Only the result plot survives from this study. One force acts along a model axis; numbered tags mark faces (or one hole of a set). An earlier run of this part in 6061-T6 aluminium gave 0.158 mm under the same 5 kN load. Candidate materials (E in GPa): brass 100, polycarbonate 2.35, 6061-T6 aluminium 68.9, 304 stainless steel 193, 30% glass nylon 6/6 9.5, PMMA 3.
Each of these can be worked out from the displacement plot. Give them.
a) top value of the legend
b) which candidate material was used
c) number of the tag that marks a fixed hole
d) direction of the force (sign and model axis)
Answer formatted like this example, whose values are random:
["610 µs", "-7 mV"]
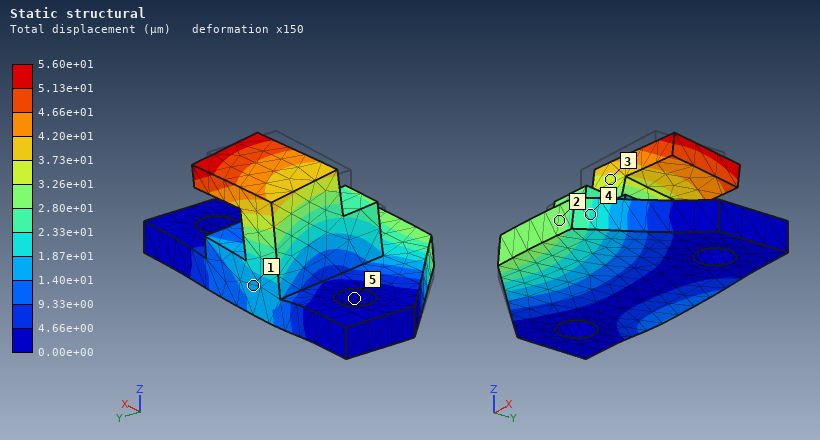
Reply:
["5.60e+01 µm", "304 stainless steel", "5", "+Y"]
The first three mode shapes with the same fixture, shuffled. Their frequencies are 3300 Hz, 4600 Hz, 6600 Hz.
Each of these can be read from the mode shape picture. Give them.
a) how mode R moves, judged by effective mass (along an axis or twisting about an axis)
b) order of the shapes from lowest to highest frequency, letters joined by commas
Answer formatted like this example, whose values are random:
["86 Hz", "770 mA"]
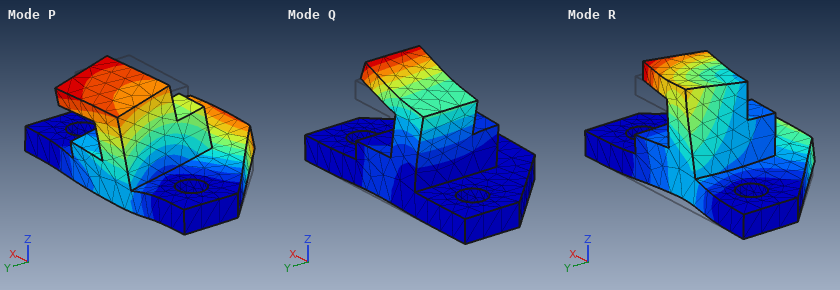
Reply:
["along Z", "P, Q, R"]
